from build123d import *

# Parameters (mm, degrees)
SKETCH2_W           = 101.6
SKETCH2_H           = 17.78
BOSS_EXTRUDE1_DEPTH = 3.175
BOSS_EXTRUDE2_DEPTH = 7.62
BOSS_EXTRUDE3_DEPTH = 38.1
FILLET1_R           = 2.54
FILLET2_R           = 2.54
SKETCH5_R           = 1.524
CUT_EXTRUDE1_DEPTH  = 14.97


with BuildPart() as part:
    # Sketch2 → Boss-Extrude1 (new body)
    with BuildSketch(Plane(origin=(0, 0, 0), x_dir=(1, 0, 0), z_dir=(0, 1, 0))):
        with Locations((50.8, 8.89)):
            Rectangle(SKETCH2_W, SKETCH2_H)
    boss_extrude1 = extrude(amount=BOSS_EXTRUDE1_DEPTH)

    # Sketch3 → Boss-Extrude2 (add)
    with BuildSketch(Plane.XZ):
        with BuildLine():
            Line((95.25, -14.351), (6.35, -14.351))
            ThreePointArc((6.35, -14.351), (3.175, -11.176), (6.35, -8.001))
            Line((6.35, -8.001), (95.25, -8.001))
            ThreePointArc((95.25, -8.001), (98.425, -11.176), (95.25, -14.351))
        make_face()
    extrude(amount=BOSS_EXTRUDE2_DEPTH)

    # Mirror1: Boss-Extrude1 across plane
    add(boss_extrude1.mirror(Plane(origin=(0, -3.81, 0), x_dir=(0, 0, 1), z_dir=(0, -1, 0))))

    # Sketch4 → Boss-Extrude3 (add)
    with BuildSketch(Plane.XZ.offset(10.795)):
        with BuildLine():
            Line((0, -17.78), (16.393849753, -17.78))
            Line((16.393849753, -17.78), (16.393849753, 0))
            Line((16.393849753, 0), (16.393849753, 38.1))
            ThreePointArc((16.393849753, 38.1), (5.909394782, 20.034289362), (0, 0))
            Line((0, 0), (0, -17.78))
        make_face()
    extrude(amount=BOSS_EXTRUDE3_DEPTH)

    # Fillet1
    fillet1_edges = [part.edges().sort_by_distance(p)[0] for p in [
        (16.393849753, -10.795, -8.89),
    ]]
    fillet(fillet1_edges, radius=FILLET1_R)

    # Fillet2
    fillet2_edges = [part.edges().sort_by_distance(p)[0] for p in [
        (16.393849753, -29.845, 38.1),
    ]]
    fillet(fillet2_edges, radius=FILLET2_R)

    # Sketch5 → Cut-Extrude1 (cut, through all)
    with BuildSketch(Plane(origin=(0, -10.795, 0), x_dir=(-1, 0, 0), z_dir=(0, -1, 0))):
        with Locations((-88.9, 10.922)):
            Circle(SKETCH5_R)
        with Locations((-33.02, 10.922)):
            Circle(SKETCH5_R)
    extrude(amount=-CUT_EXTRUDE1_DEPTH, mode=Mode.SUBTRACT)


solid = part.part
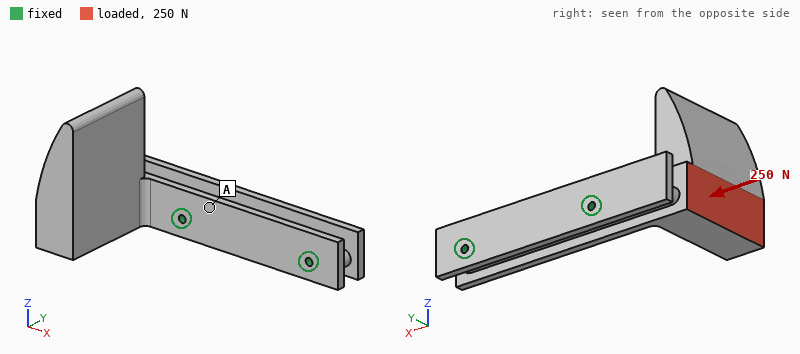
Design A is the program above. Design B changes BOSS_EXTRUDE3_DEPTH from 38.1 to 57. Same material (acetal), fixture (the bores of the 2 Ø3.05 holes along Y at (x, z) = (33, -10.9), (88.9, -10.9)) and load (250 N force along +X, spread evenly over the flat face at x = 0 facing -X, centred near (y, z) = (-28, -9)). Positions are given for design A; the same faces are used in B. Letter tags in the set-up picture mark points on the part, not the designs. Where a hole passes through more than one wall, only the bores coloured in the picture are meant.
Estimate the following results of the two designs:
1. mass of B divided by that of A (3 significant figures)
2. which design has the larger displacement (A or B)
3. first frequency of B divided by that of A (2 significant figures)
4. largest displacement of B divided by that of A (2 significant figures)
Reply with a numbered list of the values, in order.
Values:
1. 1.30
2. B
3. 0.65
4. 2.0
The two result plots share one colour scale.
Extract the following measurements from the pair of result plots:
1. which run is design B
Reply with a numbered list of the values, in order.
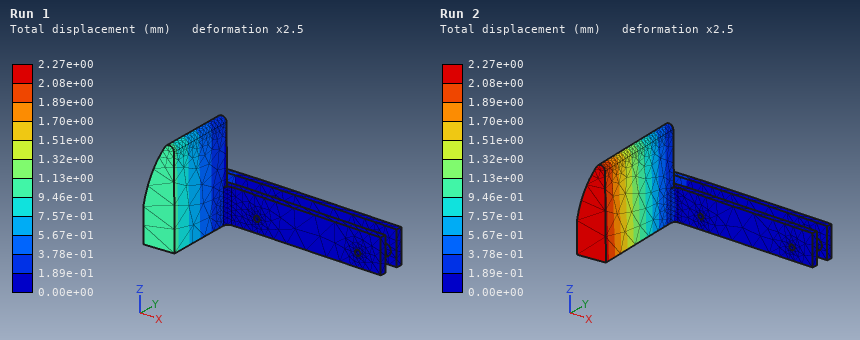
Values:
1. Run 2
